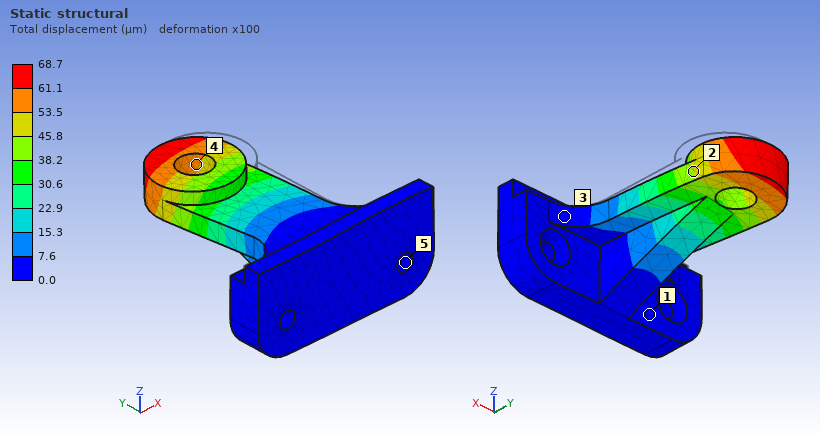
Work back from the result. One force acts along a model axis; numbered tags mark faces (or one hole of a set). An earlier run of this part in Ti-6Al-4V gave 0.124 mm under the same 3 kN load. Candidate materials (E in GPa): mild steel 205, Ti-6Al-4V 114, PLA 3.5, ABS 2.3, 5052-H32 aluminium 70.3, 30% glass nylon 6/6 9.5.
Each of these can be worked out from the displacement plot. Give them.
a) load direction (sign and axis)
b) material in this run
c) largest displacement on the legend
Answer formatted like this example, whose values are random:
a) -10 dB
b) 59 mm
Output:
a) -X
b) mild steel
c) 68.7 µm
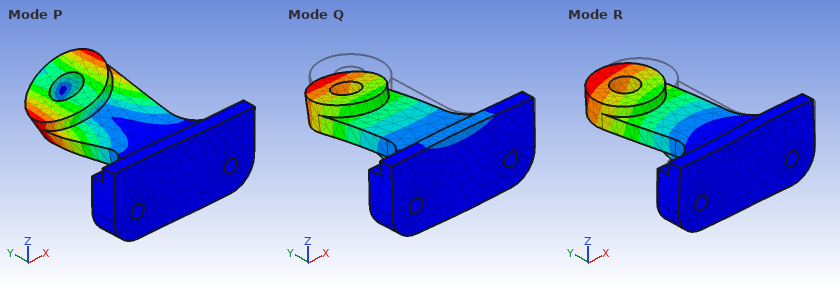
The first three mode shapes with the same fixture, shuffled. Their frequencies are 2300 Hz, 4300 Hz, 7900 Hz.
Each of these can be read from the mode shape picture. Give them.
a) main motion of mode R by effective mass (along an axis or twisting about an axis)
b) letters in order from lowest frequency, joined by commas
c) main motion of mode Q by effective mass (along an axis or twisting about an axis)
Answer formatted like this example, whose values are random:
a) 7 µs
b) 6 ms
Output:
a) along X
b) Q, R, P
c) along Z
